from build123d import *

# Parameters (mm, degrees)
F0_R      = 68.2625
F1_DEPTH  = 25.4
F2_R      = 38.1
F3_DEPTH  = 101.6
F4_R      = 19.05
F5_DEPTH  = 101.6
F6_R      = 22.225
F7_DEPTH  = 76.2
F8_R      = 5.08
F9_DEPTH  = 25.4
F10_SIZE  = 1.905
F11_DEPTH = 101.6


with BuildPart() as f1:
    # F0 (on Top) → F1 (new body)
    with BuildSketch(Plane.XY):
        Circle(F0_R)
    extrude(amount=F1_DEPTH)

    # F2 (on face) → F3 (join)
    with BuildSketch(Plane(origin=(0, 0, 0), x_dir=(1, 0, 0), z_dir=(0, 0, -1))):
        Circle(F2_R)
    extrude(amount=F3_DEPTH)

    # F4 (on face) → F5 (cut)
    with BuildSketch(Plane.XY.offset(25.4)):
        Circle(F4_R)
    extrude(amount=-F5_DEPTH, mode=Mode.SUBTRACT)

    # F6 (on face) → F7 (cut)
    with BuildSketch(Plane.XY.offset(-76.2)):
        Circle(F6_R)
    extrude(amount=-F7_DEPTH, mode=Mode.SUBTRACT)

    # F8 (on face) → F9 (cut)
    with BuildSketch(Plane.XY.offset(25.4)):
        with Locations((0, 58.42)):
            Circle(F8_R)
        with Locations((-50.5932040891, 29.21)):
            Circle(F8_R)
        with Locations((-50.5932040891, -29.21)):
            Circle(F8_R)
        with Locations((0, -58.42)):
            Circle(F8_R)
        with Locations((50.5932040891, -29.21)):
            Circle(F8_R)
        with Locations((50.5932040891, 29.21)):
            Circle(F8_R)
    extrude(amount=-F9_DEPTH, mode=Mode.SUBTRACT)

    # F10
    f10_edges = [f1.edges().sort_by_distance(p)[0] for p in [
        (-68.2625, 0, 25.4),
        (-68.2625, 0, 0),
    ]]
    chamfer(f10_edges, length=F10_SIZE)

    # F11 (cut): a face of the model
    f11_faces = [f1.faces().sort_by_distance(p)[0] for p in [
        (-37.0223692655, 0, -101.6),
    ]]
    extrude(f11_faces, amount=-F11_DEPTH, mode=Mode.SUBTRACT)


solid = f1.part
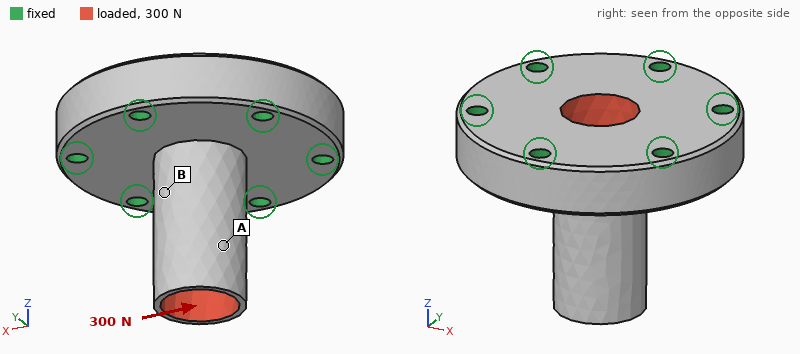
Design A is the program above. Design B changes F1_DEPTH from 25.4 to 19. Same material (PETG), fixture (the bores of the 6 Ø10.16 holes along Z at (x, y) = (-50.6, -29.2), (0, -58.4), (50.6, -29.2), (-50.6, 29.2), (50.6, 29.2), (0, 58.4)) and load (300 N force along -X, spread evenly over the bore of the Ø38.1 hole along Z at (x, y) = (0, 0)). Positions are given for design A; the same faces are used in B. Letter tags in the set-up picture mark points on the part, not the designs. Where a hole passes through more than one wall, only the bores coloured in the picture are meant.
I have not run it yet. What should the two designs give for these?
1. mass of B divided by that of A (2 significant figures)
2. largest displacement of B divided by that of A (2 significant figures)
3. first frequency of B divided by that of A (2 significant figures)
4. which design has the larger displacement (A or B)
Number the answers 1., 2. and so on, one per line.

1. 0.77
2. 1.2
3. 0.93
4. B
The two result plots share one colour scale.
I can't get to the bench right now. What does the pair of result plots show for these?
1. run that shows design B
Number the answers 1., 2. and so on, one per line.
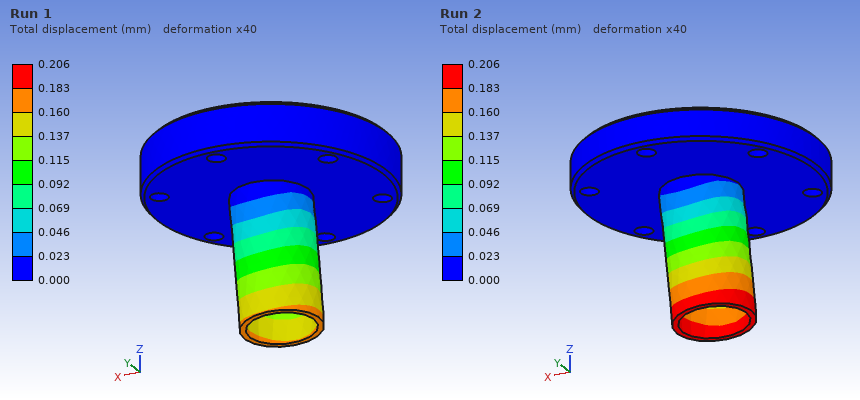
1. Run 2
